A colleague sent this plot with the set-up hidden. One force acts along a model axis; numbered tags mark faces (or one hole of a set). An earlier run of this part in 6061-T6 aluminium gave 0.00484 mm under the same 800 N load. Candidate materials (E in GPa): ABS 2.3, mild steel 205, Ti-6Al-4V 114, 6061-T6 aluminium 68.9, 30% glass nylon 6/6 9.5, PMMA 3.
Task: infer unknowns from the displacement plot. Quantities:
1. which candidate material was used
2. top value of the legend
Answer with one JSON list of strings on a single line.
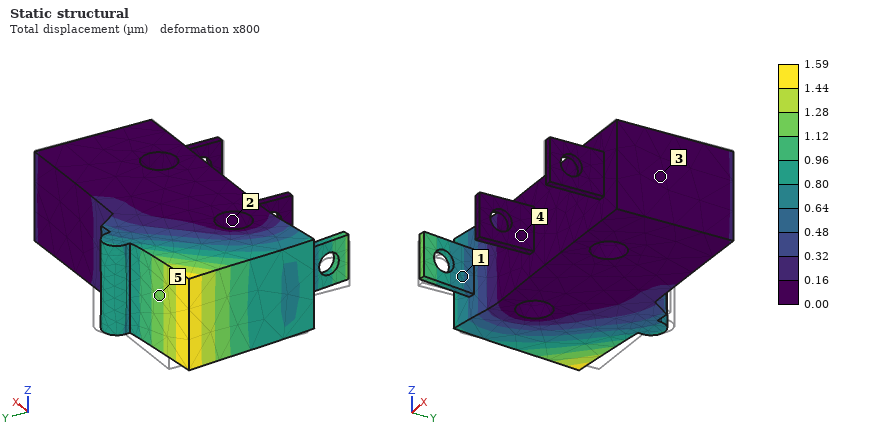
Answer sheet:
["mild steel", "1.59 µm"]
